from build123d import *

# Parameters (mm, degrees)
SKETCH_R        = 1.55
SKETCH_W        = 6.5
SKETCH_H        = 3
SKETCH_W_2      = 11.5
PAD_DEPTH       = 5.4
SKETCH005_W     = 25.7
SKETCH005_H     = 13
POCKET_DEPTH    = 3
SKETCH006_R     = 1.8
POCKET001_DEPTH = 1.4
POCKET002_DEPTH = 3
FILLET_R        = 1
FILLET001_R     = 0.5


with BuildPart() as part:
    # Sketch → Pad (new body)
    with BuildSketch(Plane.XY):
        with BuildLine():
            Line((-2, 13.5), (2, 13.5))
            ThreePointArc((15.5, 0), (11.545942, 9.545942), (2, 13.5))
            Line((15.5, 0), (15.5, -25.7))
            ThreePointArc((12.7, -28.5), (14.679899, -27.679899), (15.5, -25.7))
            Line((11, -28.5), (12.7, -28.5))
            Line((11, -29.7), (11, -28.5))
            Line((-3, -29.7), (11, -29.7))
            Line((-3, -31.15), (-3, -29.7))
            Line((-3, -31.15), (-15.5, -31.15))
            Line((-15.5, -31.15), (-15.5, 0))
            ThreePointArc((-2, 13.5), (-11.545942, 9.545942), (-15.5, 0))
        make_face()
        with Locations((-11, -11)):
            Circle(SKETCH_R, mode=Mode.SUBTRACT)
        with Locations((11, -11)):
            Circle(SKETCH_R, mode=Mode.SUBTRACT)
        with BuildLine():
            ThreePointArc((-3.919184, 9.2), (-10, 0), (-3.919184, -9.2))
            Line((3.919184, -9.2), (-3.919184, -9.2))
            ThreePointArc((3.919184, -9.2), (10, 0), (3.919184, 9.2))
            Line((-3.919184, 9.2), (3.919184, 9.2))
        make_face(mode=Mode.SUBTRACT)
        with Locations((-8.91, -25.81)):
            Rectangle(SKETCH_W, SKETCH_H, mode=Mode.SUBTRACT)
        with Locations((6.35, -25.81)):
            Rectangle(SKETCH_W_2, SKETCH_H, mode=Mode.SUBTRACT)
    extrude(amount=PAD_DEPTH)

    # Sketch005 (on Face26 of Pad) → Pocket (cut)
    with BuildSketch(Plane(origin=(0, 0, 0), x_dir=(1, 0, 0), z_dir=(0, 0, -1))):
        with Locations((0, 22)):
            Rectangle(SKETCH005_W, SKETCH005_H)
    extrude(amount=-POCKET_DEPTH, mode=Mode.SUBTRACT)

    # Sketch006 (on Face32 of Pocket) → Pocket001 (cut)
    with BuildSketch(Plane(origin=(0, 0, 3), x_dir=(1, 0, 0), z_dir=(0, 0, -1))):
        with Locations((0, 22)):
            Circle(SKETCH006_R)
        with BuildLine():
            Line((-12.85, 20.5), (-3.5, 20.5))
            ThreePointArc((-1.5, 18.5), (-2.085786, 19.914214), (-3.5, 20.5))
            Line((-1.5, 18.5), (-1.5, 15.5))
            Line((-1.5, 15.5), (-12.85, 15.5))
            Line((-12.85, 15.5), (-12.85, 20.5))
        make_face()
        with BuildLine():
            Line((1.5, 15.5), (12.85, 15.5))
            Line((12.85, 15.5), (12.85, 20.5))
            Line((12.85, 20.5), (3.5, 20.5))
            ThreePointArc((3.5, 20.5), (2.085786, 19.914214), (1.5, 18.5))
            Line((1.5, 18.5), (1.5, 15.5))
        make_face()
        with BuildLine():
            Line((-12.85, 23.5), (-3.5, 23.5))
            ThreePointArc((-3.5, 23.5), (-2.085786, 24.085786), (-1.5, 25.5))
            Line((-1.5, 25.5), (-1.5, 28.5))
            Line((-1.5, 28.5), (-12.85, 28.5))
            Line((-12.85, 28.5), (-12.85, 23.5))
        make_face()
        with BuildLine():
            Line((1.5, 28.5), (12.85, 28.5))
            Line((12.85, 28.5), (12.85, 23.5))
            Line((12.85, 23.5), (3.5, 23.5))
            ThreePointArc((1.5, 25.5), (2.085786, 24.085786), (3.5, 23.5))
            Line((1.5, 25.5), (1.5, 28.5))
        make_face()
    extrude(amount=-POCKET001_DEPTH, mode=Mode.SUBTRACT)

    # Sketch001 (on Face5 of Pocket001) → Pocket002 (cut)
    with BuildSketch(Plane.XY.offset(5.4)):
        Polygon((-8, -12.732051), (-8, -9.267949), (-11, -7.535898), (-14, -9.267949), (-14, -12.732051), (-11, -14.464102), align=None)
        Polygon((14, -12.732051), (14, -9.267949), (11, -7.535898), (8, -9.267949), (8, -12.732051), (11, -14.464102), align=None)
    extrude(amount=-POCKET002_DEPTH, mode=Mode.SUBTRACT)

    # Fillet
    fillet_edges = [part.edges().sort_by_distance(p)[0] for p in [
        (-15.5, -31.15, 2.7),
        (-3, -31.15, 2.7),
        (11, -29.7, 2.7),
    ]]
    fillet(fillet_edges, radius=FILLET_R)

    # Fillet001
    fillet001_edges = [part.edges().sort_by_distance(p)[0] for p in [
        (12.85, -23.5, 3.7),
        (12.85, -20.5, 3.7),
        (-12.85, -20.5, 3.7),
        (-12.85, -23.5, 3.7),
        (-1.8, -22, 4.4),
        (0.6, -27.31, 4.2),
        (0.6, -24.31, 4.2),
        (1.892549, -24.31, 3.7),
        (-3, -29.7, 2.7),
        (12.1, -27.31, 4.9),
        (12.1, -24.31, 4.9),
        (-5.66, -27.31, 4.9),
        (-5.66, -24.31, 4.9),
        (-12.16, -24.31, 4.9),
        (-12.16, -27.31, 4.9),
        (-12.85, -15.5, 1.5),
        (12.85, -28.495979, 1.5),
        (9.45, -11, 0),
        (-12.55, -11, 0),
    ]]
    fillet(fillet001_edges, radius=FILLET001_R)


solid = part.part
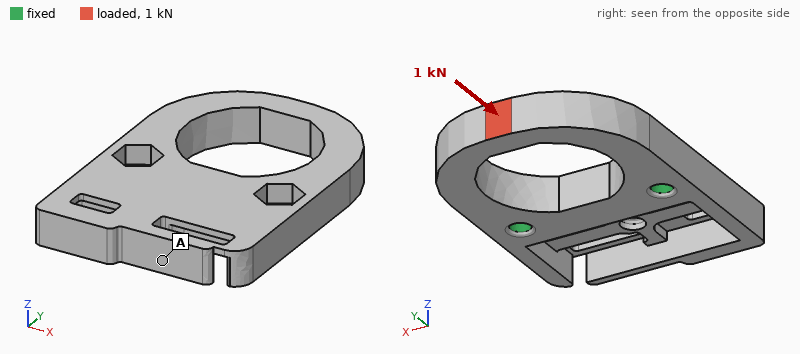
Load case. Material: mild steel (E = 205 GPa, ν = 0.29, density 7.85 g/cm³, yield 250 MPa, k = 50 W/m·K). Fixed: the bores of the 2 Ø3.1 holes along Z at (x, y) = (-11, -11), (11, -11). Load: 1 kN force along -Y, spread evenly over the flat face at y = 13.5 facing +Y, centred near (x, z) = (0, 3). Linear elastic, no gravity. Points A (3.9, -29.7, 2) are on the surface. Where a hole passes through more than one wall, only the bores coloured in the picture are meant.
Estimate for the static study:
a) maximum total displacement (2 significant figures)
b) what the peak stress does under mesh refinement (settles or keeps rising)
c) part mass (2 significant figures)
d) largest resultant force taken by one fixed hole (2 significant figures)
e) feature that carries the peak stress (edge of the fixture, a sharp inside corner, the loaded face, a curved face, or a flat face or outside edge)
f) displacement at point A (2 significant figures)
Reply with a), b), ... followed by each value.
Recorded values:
a) 18 µm
b) keeps rising
c) 28 g
d) 550 N
e) edge of the fixture
f) 3.4 µm
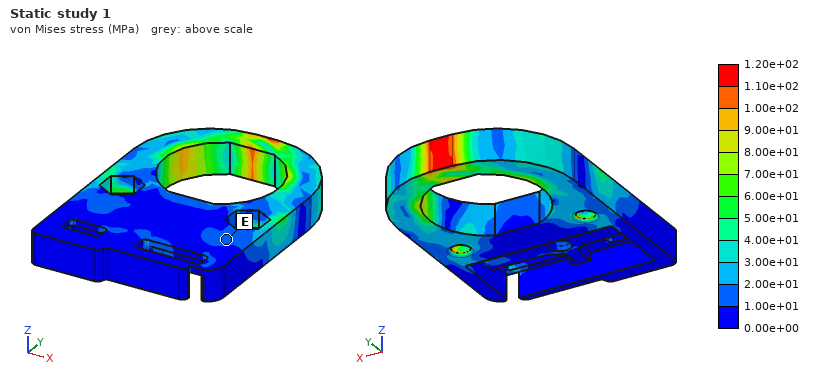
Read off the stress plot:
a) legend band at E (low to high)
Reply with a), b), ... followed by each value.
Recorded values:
a) 1.00e+01 to 2.00e+01 MPa
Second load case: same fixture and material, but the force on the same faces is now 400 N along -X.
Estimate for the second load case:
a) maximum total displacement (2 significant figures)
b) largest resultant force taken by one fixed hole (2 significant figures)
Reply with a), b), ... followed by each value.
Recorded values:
a) 12 µm
b) 410 N
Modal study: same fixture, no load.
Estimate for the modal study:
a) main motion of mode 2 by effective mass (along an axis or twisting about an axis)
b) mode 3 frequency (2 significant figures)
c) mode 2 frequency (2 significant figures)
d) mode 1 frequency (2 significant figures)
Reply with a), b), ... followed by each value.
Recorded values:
a) along Z
b) 9300 Hz
c) 6700 Hz
d) 4300 Hz
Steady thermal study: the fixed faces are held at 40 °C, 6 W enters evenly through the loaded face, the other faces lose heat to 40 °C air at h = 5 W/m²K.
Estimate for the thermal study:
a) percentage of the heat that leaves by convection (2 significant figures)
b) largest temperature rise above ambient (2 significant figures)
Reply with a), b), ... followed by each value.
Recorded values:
a) 3.4 %
b) 69 K
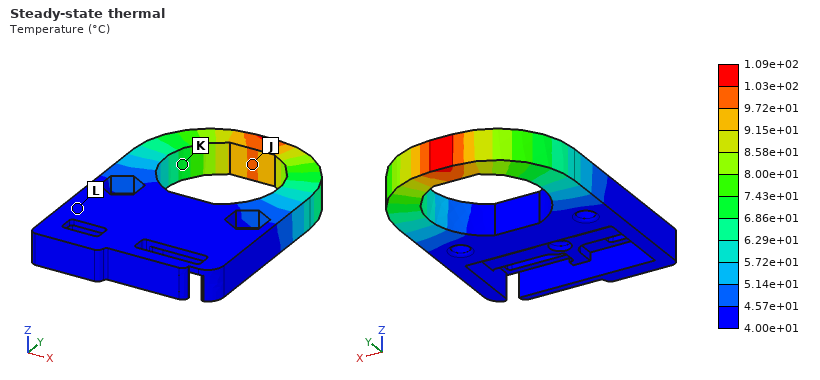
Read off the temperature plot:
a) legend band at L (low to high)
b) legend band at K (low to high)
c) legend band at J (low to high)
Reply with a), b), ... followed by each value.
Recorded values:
a) 4.00e+01 to 4.57e+01 °C
b) 6.86e+01 to 7.43e+01 °C
c) 9.72e+01 to 1.03e+02 °C
